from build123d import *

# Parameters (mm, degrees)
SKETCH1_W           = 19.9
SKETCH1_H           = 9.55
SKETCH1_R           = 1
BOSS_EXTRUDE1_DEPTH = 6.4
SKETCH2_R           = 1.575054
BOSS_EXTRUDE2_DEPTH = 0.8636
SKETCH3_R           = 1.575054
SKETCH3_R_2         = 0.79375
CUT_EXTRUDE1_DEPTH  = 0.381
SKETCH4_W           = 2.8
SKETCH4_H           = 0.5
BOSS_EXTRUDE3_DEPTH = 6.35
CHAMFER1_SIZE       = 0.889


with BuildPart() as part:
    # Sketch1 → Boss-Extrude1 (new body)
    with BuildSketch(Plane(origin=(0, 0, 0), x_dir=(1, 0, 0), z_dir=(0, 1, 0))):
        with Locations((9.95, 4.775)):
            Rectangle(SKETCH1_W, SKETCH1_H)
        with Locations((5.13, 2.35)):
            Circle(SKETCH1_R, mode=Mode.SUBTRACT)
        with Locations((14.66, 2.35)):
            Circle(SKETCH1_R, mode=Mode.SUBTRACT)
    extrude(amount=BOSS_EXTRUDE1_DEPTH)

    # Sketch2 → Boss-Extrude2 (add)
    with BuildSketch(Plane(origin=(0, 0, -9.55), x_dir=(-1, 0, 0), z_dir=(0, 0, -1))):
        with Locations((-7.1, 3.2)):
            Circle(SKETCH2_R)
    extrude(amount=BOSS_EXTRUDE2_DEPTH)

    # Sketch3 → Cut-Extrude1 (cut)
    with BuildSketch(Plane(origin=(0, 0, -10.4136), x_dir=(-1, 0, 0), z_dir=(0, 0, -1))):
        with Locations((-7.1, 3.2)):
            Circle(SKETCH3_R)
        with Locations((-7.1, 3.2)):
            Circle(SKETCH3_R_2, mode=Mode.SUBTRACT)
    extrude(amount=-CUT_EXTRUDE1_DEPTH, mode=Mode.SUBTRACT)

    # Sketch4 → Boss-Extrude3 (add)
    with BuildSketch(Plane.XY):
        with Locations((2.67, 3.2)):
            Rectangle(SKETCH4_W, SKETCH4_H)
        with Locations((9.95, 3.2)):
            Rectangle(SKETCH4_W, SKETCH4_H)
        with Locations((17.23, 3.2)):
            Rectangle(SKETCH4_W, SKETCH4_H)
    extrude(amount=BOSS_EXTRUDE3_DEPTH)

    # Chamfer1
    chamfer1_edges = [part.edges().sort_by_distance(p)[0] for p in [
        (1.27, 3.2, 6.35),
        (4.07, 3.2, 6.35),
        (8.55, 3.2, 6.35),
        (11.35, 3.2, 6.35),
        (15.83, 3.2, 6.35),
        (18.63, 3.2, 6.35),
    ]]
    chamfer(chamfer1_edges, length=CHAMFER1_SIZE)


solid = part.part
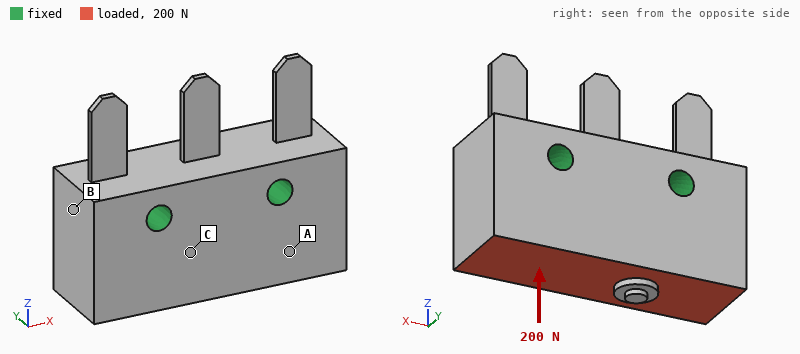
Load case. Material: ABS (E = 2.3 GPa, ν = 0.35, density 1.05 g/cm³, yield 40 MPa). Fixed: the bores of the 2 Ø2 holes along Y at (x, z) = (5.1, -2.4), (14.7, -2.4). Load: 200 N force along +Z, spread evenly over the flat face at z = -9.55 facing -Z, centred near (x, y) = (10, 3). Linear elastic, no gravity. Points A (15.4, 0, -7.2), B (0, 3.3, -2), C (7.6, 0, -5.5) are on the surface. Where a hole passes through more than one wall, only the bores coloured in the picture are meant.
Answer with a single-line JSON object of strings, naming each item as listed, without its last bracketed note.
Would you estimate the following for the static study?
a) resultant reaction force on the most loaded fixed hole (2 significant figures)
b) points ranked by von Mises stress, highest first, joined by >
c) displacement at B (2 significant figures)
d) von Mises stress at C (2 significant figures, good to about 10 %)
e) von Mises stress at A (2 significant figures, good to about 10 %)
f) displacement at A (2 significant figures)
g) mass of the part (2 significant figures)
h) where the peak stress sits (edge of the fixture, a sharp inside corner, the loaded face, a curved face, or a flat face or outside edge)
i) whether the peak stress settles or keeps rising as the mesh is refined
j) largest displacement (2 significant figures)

{"resultant reaction force on the most loaded fixed hole": "100 N", "points ranked by von Mises stress, highest first, joined by >": "A > C > B", "displacement at B": "6.3 µm", "von Mises stress at C": "1.3 MPa", "von Mises stress at A": "2.2 MPa", "displacement at A": "5.6 µm", "mass of the part": "1.3 g", "where the peak stress sits": "edge of the fixture", "whether the peak stress settles or keeps rising as the mesh is refined": "keeps rising", "largest displacement": "13 µm"}
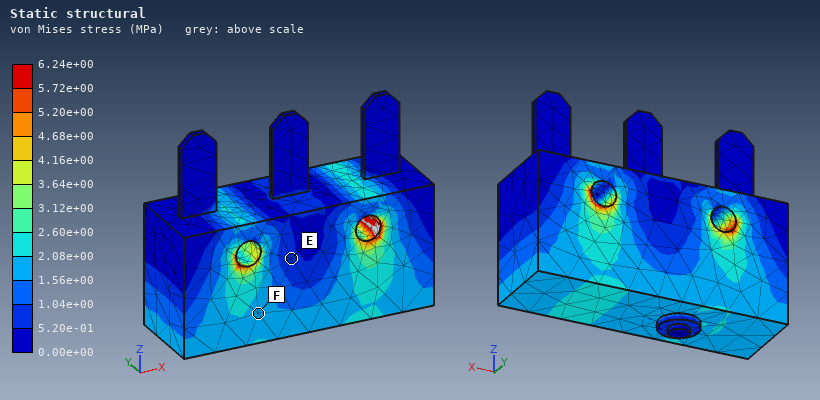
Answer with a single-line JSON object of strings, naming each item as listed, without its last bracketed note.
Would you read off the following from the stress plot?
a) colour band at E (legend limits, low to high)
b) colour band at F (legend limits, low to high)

{"colour band at E": "5.20e-01 to 1.04e+00 MPa", "colour band at F": "1.56e+00 to 2.08e+00 MPa"}
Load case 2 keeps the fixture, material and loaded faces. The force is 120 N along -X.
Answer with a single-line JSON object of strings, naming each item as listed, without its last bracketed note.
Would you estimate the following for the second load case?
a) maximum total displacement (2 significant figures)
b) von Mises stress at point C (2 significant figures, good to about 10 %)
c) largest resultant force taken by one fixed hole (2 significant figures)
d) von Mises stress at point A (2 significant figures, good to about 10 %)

{"maximum total displacement": "26 µm", "von Mises stress at point C": "3.3 MPa", "largest resultant force taken by one fixed hole": "94 N", "von Mises stress at point A": "1.6 MPa"}
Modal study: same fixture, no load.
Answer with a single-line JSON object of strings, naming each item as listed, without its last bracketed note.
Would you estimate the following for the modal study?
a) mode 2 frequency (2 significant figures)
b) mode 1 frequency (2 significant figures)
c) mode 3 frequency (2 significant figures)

{"mode 2 frequency": "3200 Hz", "mode 1 frequency": "3200 Hz", "mode 3 frequency": "3200 Hz"}
